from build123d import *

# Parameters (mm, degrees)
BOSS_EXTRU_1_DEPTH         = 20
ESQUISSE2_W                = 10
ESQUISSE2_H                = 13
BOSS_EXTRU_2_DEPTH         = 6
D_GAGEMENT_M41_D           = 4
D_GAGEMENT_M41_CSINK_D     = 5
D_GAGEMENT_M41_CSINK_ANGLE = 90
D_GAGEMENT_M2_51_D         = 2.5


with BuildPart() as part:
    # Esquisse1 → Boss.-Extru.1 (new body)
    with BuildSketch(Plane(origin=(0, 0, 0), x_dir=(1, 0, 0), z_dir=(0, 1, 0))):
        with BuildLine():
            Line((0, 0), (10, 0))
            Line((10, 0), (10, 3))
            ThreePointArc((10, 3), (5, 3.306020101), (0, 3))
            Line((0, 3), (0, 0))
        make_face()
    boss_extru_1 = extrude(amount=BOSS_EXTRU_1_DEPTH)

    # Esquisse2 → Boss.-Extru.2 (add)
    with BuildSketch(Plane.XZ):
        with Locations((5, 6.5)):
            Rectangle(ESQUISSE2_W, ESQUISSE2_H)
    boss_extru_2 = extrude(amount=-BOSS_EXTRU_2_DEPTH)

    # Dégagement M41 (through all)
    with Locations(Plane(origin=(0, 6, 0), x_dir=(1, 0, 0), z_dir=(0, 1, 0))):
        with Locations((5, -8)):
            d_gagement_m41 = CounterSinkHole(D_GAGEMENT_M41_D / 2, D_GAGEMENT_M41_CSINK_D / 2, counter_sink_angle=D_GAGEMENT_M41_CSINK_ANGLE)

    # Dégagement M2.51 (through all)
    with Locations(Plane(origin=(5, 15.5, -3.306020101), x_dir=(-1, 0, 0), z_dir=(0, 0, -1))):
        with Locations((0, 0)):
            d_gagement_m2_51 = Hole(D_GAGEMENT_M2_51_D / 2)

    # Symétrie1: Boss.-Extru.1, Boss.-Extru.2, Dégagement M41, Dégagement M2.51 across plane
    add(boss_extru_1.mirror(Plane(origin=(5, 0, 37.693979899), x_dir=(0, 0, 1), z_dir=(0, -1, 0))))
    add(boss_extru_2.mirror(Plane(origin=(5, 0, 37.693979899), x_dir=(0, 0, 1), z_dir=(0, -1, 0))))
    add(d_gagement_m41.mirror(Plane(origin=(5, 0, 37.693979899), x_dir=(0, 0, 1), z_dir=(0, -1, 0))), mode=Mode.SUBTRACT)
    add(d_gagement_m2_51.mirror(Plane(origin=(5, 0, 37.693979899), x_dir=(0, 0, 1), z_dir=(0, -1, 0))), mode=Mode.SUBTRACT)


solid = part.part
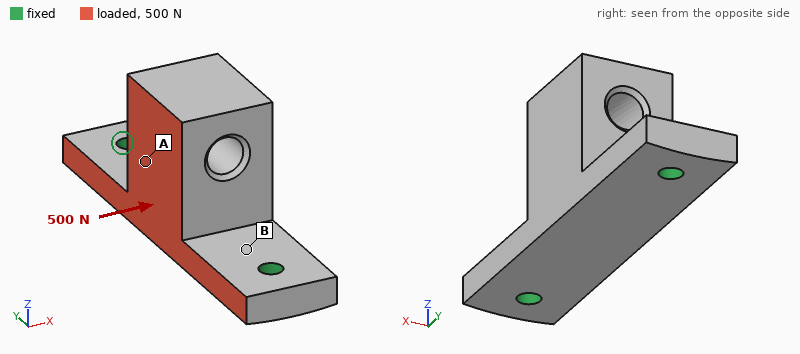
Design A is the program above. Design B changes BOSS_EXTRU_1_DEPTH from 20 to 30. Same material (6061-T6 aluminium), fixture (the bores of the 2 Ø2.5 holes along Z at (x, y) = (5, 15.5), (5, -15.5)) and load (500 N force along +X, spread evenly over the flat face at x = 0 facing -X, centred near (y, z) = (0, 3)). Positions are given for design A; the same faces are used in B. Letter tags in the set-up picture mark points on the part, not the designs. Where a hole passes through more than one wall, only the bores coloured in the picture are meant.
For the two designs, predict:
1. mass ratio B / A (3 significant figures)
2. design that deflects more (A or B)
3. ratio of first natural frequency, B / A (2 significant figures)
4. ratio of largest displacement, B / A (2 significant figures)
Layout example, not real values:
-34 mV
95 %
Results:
1.24
A
1.0
0.80
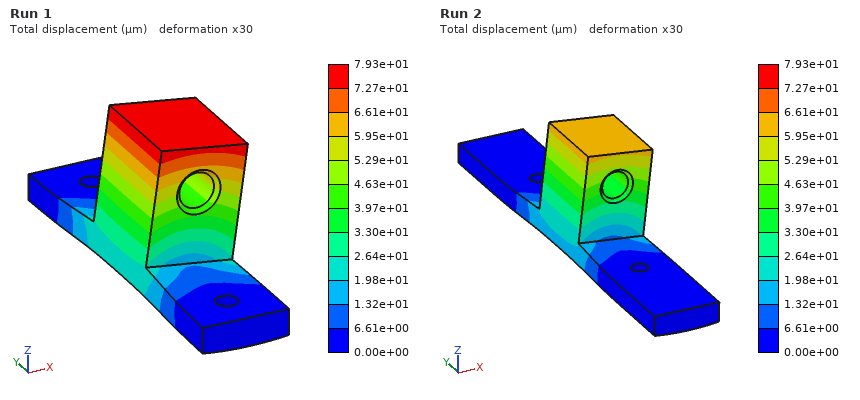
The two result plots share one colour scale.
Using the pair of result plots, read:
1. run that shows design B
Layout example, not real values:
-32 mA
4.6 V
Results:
Run 2
